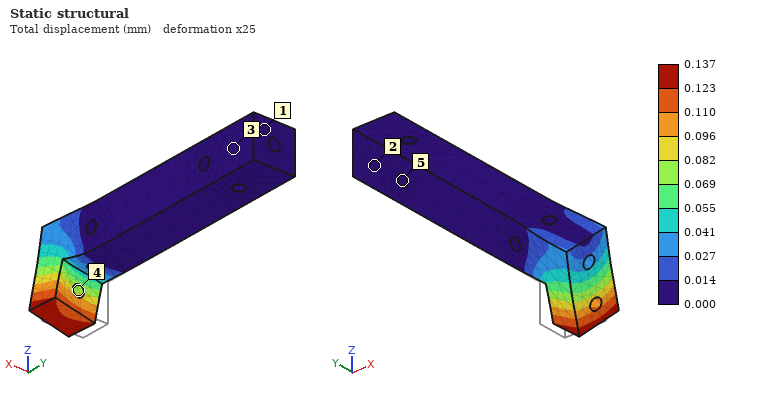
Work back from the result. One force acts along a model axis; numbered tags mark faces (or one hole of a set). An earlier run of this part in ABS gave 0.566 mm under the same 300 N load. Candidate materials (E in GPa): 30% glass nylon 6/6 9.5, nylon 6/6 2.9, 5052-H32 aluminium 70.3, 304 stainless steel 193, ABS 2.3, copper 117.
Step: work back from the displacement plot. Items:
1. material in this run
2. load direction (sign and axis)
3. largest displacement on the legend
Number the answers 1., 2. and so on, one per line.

1. 30% glass nylon 6/6
2. +X
3. 0.137 mm
